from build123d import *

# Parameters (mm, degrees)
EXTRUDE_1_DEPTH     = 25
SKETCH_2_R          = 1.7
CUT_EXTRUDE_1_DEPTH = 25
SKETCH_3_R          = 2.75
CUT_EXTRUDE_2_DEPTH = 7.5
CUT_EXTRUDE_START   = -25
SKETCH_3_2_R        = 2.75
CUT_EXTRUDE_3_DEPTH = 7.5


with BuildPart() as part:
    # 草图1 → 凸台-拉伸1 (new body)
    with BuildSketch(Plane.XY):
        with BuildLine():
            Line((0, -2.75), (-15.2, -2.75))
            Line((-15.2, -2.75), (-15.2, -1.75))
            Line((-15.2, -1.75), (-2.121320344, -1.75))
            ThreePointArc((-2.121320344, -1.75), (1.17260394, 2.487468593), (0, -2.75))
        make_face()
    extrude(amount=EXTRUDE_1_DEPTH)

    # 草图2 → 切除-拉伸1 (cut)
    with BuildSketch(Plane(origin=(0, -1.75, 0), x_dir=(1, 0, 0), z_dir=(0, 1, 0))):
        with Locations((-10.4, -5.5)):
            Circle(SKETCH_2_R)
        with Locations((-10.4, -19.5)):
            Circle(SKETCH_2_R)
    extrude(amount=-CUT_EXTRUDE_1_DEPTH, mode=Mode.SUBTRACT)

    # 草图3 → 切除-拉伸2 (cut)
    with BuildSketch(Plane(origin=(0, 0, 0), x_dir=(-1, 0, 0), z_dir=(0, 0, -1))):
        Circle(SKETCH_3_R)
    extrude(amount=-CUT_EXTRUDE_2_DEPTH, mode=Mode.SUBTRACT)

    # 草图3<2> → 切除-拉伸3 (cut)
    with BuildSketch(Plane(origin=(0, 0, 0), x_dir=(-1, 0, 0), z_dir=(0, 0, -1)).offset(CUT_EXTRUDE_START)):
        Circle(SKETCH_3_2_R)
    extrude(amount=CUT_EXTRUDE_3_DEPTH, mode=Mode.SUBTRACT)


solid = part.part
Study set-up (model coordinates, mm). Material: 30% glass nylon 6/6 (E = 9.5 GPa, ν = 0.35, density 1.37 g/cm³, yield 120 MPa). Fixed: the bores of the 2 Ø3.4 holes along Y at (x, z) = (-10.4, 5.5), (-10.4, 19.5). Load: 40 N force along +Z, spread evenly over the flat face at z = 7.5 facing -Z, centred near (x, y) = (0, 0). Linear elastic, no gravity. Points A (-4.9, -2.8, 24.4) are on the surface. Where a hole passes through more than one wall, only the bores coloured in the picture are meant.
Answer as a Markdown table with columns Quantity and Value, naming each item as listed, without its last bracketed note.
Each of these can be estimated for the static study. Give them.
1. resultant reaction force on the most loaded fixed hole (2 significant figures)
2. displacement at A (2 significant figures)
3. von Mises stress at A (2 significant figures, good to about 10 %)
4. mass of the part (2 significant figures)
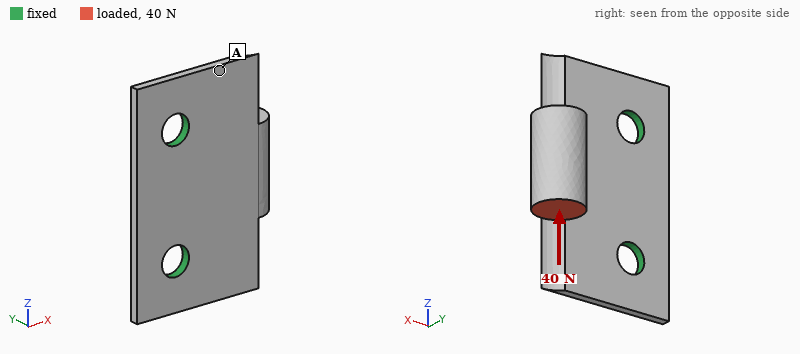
| Quantity | Value |
|---|---|
| resultant reaction force on the most loaded fixed hole | 33 N |
| displacement at A | 24 µm |
| von Mises stress at A | 4.3 MPa |
| mass of the part | 0.77 g |
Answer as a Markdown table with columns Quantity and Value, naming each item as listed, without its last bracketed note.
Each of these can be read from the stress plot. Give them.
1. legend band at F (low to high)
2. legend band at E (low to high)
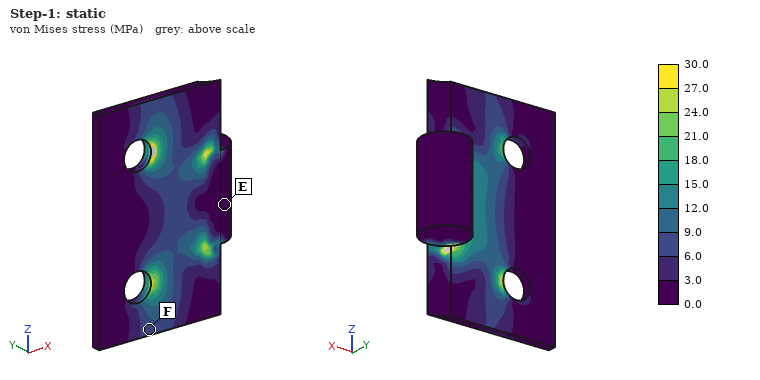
| Quantity | Value |
|---|---|
| legend band at F | 6.0 to 9.0 MPa |
| legend band at E | 0.0 to 3.0 MPa |
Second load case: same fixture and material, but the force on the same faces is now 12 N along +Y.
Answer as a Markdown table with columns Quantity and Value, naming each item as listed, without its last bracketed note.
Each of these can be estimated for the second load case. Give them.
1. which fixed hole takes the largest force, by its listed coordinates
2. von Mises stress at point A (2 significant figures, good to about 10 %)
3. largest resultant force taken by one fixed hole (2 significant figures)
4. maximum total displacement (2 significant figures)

| Quantity | Value |
|---|---|
| which fixed hole takes the largest force, by its listed coordinates | (-10.4, 5.5) |
| von Mises stress at point A | 8.5 MPa |
| largest resultant force taken by one fixed hole | 11 N |
| maximum total displacement | 0.33 mm |
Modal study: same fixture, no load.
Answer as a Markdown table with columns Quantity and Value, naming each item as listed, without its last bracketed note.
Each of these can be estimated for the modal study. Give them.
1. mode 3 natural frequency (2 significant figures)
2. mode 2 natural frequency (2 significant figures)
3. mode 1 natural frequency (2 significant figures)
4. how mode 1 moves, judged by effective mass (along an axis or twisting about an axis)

| Quantity | Value |
|---|---|
| mode 3 natural frequency | 8000 Hz |
| mode 2 natural frequency | 5600 Hz |
| mode 1 natural frequency | 1900 Hz |
| how mode 1 moves, judged by effective mass | along Y |
